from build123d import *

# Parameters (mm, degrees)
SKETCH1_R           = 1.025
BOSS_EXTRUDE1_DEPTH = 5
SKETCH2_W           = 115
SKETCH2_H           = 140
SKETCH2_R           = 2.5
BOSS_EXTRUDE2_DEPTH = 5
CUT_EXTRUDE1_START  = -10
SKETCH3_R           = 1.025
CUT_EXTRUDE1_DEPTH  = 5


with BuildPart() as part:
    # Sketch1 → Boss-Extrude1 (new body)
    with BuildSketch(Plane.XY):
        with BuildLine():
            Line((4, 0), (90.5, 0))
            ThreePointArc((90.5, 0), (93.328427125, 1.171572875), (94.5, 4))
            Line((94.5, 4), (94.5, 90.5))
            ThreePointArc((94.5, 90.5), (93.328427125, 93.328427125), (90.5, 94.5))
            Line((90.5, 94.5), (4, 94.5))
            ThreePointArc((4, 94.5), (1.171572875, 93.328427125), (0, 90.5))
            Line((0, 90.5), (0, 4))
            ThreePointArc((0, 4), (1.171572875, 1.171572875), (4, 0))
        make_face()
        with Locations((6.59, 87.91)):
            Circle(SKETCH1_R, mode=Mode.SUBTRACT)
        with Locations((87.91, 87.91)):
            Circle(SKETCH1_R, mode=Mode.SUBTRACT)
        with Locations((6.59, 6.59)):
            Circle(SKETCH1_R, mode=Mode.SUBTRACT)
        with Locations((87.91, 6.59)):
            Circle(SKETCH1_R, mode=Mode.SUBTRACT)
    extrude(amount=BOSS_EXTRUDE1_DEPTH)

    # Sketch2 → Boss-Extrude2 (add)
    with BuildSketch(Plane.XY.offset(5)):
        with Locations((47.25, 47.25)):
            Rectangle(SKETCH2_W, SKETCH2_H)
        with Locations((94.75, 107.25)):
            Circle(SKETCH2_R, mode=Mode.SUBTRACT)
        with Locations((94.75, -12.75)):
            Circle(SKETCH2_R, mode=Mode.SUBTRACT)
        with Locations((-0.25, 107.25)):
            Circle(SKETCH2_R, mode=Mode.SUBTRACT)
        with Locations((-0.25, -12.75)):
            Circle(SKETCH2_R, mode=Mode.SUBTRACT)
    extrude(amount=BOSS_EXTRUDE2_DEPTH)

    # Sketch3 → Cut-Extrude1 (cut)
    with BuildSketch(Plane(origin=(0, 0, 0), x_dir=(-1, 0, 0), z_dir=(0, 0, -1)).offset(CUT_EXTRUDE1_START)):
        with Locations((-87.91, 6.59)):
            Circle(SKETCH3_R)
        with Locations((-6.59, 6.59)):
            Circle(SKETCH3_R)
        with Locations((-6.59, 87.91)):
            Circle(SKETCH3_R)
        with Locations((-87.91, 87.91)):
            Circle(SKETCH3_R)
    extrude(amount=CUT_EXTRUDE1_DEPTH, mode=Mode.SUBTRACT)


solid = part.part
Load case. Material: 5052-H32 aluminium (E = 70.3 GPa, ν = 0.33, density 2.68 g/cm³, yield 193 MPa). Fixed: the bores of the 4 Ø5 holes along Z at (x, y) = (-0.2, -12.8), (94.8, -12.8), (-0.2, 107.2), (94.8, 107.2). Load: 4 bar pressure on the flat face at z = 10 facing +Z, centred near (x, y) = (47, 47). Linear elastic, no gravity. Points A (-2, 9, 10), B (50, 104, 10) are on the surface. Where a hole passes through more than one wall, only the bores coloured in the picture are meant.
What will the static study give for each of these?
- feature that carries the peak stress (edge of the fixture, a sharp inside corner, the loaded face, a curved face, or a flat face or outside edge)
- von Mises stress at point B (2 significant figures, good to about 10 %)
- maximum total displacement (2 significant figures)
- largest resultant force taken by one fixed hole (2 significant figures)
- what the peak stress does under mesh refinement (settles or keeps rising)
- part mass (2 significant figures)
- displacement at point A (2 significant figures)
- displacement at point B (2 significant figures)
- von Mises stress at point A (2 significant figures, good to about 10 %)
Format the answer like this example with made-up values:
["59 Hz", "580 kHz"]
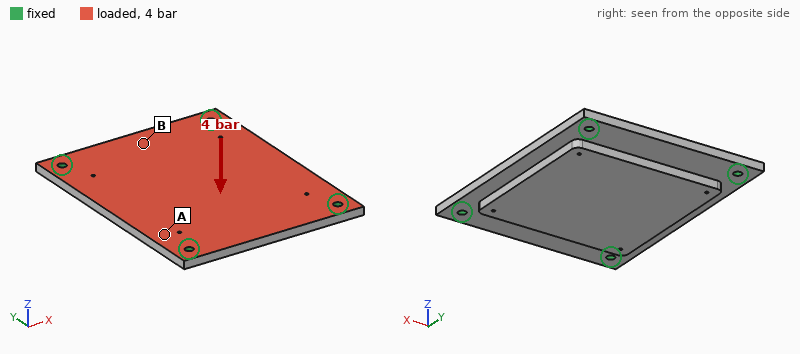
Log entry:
["edge of the fixture", "24 MPa", "0.16 mm", "2.4 kN", "keeps rising", "330 g", "0.072 mm", "0.100 mm", "14 MPa"]
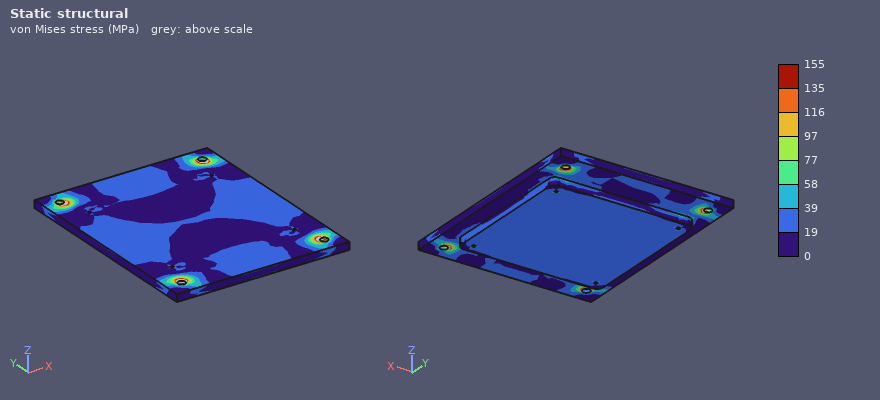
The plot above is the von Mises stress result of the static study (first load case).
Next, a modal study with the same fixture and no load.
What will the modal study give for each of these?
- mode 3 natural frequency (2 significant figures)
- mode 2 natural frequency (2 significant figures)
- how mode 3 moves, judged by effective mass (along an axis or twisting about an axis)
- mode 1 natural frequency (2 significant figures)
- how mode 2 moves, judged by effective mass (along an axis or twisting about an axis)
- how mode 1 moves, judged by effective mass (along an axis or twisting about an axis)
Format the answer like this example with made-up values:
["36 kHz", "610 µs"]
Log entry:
["3600 Hz", "3000 Hz", "twisting about X", "1900 Hz", "twisting about Y", "along Z"]
